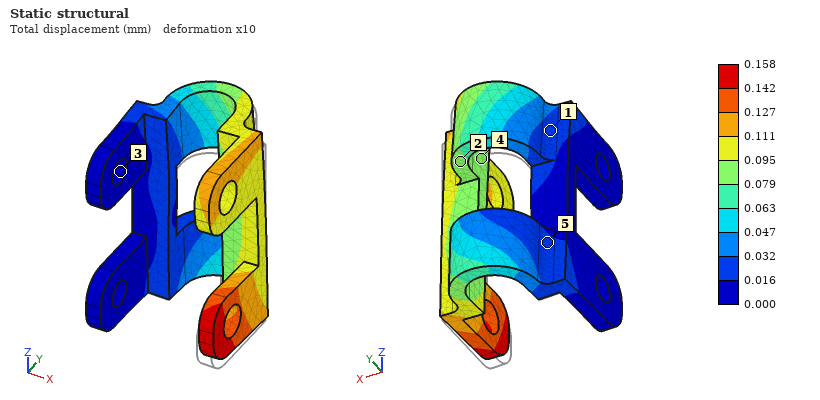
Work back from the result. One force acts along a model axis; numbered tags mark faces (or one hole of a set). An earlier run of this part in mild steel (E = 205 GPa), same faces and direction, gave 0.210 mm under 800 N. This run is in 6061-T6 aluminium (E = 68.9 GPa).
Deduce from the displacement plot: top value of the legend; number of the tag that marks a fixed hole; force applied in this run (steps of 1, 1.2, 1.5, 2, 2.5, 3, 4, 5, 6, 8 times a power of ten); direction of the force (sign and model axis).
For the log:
0.158 mm
3
200 N
+Z
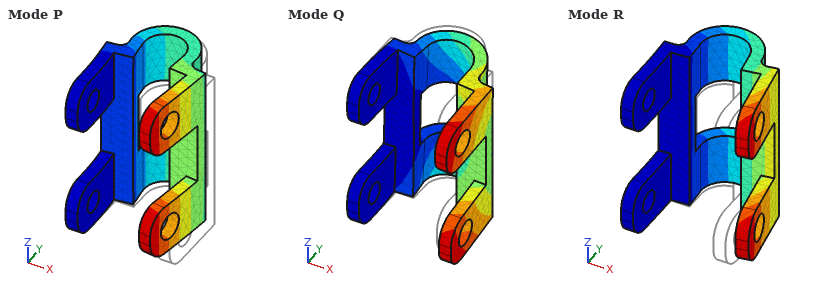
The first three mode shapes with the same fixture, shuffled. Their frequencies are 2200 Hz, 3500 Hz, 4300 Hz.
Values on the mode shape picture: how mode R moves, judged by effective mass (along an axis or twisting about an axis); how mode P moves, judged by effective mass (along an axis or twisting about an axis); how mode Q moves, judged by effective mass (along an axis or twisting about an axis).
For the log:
along Y
along X
along Z
